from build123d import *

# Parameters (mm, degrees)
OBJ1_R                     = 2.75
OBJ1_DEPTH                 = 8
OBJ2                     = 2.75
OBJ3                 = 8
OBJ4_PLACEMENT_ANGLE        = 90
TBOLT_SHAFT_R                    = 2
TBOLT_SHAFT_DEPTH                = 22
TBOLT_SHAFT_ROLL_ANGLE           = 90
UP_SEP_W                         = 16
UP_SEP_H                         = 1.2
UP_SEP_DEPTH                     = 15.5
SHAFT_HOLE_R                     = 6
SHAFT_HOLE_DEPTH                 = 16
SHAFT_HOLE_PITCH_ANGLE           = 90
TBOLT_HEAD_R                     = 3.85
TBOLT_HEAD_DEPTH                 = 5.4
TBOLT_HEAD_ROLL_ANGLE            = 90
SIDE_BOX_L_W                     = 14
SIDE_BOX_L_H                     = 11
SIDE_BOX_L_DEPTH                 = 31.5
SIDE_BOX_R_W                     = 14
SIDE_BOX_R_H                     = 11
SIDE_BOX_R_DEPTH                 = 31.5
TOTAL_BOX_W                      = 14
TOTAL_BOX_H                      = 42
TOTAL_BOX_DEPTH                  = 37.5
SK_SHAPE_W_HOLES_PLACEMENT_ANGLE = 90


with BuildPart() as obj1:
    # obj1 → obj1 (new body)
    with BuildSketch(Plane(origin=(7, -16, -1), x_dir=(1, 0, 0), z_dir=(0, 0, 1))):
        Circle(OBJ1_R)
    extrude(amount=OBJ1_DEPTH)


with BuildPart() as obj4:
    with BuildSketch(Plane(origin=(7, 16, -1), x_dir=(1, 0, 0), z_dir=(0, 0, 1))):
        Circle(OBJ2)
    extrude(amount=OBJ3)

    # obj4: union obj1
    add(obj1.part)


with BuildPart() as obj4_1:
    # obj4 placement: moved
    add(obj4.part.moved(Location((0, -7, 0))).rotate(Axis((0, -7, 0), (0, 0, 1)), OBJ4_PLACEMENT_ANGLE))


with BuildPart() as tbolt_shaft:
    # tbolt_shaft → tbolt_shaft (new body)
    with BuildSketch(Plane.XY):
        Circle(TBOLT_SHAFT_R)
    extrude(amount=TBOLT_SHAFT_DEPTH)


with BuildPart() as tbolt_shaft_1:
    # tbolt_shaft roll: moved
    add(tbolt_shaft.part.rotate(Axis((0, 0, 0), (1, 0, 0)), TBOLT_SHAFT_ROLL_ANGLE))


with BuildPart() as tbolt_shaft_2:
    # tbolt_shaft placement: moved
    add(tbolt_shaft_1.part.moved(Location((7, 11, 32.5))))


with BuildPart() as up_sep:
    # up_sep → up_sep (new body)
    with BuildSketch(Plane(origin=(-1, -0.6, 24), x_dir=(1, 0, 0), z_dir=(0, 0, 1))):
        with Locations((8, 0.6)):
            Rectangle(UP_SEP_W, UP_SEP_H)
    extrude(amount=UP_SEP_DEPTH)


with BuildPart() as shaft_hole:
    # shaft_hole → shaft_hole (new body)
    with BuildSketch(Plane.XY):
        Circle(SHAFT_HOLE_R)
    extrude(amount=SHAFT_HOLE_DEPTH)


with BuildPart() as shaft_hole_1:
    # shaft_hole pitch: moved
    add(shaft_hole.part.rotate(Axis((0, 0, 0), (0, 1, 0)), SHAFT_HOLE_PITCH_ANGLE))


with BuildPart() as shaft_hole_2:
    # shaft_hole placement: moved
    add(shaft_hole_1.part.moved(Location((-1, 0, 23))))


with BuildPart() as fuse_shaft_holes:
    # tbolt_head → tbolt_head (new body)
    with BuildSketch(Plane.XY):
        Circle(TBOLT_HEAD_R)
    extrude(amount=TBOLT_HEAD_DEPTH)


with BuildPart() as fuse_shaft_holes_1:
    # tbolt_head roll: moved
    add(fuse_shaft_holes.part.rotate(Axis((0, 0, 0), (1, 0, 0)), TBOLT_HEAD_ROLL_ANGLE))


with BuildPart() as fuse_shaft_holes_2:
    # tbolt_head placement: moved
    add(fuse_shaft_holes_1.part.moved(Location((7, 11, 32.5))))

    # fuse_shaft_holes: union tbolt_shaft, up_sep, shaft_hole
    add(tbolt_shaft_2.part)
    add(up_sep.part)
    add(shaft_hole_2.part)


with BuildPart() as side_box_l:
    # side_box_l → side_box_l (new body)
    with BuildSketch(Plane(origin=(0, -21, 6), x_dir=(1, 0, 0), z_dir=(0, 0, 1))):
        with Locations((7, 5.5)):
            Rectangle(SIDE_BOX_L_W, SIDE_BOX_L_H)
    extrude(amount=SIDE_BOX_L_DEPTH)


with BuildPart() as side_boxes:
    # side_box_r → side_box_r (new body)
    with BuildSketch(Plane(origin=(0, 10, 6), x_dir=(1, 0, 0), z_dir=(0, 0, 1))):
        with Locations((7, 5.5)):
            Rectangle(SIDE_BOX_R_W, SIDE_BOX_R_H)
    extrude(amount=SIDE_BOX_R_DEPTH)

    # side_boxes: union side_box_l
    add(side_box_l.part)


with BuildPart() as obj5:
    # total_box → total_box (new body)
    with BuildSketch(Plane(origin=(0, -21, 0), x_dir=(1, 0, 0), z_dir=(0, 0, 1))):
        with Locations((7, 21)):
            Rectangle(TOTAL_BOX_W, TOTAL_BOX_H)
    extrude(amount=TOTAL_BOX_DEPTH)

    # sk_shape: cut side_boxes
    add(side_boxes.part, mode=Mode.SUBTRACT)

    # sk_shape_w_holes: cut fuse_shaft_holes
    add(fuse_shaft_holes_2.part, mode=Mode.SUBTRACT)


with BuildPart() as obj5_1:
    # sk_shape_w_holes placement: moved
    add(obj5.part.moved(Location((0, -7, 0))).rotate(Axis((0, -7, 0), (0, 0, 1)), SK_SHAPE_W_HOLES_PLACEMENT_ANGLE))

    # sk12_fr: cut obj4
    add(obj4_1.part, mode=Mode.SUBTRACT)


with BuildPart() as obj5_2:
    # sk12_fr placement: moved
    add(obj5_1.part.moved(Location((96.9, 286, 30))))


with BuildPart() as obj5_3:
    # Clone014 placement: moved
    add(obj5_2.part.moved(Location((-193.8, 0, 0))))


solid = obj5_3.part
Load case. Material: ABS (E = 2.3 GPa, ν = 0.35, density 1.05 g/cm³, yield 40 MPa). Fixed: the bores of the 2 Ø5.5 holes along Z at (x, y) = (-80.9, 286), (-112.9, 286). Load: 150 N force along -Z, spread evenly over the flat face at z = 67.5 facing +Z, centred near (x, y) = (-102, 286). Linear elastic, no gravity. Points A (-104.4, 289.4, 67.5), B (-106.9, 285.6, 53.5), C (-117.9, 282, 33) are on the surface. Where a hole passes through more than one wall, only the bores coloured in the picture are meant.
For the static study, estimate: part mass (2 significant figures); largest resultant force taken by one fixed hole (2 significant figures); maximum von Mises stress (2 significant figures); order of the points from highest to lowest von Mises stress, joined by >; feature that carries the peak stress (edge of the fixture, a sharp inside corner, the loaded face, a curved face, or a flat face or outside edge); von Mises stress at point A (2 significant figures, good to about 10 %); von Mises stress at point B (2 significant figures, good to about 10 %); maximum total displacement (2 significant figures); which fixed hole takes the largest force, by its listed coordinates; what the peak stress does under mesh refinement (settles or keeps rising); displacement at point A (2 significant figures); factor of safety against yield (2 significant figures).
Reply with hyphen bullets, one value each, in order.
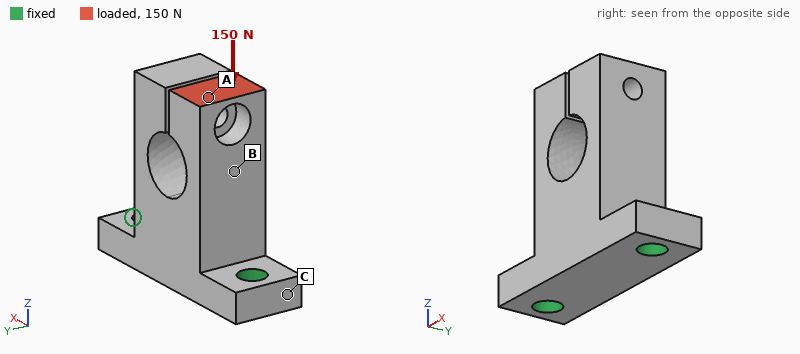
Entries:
- 10 g
- 110 N
- 15 MPa
- B > A > C
- a curved face
- 2.4 MPa
- 6.3 MPa
- 0.28 mm
- (-112.9, 286)
- settles
- 0.23 mm
- 2.7
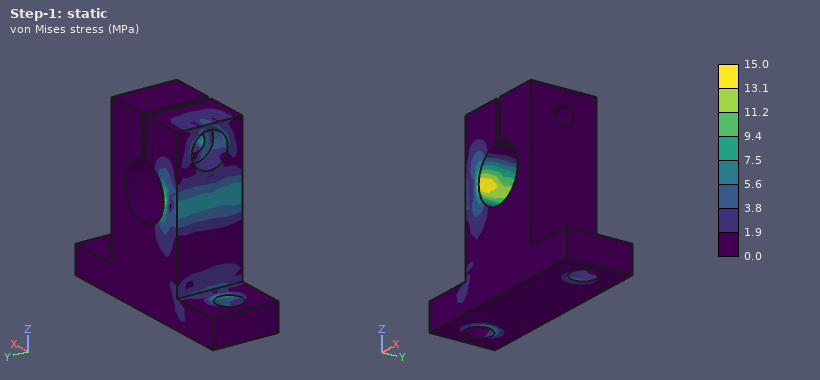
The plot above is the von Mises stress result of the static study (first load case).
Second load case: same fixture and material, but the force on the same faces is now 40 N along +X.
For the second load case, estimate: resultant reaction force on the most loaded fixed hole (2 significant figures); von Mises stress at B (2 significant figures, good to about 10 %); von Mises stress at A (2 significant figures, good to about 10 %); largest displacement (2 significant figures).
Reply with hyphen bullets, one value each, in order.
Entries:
- 64 N
- 12 MPa
- 1.2 MPa
- 0.58 mm
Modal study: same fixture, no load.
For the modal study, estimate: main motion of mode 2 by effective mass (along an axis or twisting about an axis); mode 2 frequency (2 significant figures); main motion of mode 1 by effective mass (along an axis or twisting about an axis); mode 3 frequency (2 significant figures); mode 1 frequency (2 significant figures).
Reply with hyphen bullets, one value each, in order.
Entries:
- along X
- 1600 Hz
- along Y
- 1800 Hz
- 1300 Hz
